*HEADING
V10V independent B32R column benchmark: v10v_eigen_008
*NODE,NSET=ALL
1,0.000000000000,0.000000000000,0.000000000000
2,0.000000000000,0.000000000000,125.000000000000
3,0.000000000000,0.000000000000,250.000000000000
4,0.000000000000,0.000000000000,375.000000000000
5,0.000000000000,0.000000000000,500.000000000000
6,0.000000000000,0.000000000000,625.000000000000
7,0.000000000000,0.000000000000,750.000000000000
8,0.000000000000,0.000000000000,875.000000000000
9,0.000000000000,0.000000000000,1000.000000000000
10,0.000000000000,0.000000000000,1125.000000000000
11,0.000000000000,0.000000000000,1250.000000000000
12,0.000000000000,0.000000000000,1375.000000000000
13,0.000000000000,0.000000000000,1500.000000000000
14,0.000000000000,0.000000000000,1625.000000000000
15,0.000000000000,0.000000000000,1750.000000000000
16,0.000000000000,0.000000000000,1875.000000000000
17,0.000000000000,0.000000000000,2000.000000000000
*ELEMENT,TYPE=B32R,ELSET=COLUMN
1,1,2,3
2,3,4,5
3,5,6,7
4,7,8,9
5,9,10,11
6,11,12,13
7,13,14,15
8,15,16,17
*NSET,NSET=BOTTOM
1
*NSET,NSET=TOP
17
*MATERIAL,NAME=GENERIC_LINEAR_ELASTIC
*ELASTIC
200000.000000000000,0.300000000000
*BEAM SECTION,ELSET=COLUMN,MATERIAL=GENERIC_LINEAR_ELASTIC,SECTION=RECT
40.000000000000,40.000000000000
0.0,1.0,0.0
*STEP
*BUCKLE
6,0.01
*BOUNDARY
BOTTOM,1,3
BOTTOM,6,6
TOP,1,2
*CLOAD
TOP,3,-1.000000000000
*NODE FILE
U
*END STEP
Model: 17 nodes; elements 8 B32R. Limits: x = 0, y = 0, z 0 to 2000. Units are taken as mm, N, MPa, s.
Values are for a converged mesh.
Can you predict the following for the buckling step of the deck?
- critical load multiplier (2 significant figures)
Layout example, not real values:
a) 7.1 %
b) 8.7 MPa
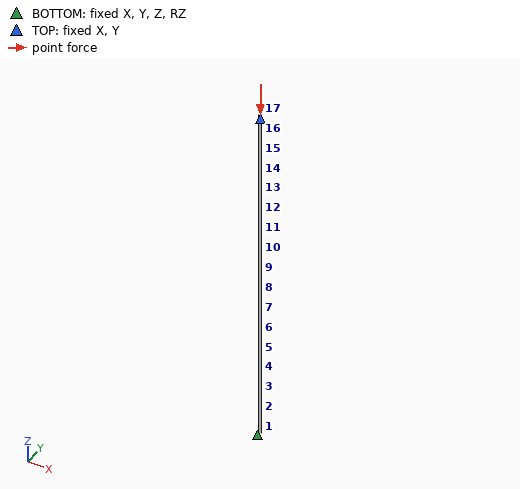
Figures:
a) 1.1e+05
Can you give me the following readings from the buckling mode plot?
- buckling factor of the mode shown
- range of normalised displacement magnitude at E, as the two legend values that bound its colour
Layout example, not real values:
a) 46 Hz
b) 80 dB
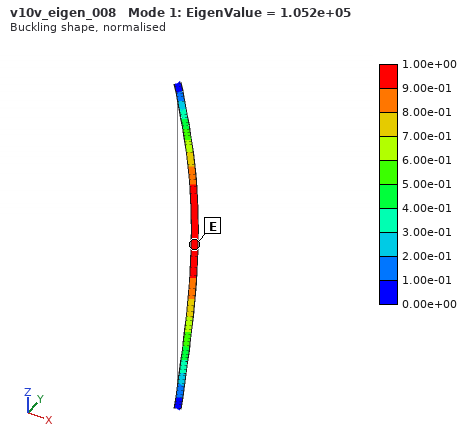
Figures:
a) 1.052e+05
b) 9.00e-01 to 1.00e+00
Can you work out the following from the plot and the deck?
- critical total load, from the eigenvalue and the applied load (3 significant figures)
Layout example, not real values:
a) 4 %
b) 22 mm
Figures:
a) 1.05e+05 N
